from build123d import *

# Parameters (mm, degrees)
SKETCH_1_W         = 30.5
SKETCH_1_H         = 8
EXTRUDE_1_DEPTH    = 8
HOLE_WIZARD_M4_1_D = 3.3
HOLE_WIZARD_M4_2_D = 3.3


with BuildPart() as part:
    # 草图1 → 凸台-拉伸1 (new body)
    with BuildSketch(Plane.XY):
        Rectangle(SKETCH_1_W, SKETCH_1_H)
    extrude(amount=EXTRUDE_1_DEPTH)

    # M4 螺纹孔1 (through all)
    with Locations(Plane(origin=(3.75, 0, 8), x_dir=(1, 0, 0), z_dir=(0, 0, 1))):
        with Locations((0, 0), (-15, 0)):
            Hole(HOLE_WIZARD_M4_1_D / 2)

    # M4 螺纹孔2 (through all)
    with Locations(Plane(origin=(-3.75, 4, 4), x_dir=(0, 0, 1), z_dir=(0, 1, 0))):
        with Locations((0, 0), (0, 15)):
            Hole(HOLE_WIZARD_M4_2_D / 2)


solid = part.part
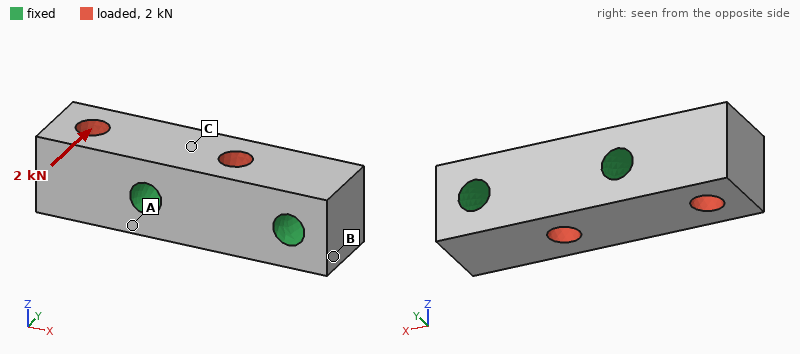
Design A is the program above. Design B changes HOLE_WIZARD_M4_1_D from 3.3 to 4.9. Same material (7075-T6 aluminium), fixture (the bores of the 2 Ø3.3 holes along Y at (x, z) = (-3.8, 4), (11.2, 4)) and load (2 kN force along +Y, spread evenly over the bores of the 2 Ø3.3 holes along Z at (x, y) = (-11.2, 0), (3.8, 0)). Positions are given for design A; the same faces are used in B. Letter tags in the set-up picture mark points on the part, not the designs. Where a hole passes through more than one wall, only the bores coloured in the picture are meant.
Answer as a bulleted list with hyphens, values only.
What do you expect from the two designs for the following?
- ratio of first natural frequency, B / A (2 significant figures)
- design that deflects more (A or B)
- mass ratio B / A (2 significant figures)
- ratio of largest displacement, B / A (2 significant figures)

- 0.98
- B
- 0.90
- 1.6
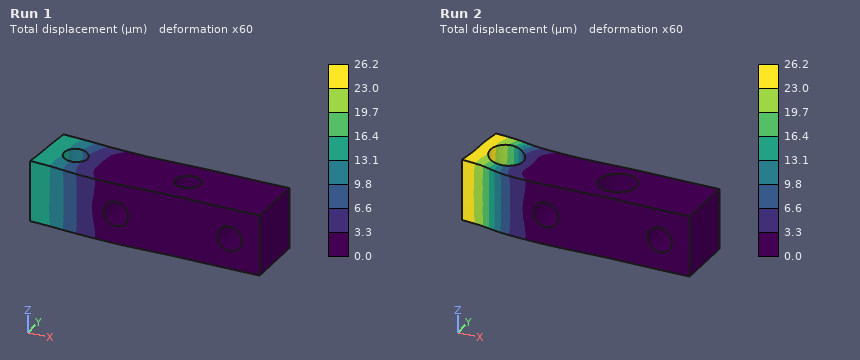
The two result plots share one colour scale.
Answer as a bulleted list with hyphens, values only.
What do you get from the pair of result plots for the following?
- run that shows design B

- Run 2
